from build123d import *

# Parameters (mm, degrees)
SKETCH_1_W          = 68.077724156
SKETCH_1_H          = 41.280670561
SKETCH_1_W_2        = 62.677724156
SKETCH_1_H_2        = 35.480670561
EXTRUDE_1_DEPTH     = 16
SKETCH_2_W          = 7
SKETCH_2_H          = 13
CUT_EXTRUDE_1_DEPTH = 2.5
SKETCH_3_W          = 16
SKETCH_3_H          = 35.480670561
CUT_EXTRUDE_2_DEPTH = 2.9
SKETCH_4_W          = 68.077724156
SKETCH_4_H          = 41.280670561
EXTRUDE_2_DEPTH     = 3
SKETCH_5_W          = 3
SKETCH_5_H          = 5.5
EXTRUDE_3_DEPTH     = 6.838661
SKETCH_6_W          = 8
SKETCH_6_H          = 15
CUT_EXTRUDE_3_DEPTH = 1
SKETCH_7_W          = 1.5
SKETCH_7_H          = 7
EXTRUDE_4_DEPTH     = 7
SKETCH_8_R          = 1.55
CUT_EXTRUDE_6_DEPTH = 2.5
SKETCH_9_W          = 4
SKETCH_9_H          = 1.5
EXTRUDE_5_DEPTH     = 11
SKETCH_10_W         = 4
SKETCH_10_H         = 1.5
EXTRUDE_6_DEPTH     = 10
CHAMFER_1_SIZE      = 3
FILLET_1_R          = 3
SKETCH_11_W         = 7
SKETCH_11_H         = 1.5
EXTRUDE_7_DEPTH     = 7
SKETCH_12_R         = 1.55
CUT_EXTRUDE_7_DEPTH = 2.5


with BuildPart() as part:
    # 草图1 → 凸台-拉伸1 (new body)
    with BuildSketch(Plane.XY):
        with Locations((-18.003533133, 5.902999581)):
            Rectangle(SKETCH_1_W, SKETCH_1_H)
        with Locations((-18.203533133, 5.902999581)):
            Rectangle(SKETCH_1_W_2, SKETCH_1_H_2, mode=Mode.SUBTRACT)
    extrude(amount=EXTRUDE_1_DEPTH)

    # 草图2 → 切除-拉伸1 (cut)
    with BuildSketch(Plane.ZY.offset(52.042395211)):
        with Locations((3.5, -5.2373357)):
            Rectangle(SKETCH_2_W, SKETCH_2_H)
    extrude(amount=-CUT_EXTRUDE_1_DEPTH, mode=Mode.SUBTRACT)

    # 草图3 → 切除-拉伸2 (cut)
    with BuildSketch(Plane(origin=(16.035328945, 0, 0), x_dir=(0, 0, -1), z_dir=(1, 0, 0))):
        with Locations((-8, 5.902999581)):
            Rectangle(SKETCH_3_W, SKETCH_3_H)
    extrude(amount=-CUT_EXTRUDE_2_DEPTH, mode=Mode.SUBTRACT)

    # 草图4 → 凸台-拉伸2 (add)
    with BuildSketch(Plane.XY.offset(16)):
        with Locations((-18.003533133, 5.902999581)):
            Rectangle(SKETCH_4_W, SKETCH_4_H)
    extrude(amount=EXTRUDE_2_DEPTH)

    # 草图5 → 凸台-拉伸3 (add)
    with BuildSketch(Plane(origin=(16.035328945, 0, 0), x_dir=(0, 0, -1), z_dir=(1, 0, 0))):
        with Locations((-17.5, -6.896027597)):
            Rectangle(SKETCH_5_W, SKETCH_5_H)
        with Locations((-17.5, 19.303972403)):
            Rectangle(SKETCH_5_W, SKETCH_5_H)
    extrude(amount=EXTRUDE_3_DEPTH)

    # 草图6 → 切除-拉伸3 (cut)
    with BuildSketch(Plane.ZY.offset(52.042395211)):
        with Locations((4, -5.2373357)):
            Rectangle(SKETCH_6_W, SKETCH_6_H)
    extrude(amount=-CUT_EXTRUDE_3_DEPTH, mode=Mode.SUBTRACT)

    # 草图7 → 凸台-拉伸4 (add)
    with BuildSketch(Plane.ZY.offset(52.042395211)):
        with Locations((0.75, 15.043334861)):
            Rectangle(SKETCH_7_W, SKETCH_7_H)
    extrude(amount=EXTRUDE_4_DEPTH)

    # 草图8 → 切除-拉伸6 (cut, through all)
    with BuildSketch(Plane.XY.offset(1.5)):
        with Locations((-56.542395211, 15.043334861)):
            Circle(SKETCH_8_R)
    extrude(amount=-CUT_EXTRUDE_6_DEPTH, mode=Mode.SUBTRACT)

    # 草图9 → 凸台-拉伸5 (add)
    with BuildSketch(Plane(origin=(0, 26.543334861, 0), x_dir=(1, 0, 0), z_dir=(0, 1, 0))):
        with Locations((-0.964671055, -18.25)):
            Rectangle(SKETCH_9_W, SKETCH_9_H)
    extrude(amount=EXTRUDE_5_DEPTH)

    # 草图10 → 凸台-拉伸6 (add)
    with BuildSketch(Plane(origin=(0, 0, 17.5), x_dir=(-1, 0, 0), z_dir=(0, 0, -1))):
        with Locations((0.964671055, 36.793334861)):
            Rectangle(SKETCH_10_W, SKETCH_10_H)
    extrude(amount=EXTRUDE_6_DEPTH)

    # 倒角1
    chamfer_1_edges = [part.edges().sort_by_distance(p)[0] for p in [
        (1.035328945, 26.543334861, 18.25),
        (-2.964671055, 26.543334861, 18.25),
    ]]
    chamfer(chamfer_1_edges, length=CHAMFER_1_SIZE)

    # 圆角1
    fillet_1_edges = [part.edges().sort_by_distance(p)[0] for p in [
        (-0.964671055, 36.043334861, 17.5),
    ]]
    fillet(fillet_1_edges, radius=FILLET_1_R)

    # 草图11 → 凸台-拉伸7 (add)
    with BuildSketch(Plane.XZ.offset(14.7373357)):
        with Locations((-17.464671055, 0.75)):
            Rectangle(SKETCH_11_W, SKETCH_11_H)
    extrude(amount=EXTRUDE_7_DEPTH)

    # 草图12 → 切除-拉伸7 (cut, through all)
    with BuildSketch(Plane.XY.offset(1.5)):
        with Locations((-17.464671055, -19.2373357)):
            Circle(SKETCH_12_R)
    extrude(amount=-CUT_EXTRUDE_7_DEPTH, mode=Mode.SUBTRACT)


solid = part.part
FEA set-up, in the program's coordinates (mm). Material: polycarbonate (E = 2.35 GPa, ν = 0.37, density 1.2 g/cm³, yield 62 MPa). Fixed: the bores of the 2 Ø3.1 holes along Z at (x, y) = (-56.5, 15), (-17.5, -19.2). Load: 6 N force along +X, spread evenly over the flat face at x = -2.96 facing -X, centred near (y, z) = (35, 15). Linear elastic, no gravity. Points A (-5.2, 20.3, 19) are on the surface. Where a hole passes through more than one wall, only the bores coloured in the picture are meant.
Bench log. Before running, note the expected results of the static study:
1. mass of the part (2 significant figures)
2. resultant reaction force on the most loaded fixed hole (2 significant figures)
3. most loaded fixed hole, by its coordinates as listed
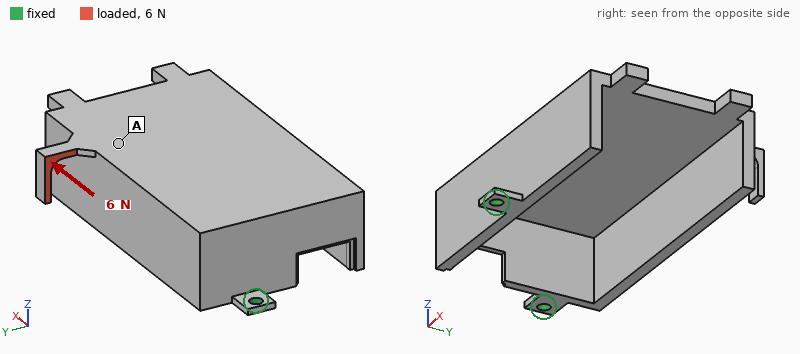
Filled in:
20 g
6.9 N
(-56.5, 15)
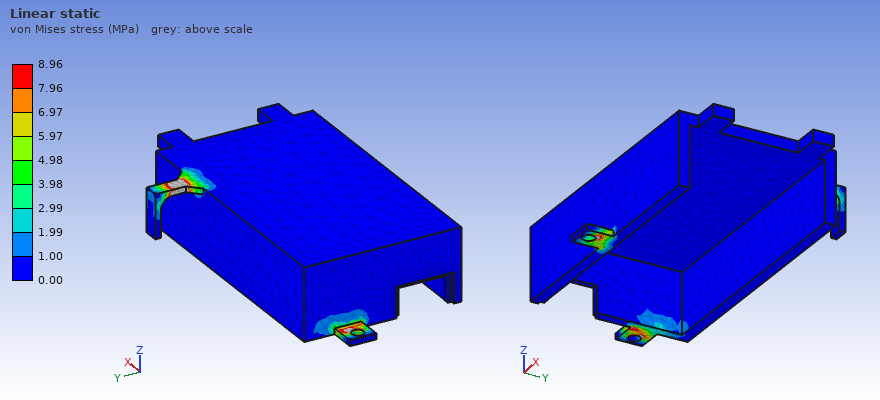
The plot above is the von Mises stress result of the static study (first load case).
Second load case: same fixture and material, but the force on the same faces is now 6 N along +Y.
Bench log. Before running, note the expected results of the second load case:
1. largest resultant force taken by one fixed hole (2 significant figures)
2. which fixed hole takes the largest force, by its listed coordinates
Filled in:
6.1 N
(-17.5, -19.2)
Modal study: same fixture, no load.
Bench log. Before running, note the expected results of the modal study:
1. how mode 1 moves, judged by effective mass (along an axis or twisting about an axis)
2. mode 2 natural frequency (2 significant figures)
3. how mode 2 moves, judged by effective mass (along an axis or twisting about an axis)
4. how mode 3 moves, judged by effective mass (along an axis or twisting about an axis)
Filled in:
along Z
370 Hz
along Y
along X
